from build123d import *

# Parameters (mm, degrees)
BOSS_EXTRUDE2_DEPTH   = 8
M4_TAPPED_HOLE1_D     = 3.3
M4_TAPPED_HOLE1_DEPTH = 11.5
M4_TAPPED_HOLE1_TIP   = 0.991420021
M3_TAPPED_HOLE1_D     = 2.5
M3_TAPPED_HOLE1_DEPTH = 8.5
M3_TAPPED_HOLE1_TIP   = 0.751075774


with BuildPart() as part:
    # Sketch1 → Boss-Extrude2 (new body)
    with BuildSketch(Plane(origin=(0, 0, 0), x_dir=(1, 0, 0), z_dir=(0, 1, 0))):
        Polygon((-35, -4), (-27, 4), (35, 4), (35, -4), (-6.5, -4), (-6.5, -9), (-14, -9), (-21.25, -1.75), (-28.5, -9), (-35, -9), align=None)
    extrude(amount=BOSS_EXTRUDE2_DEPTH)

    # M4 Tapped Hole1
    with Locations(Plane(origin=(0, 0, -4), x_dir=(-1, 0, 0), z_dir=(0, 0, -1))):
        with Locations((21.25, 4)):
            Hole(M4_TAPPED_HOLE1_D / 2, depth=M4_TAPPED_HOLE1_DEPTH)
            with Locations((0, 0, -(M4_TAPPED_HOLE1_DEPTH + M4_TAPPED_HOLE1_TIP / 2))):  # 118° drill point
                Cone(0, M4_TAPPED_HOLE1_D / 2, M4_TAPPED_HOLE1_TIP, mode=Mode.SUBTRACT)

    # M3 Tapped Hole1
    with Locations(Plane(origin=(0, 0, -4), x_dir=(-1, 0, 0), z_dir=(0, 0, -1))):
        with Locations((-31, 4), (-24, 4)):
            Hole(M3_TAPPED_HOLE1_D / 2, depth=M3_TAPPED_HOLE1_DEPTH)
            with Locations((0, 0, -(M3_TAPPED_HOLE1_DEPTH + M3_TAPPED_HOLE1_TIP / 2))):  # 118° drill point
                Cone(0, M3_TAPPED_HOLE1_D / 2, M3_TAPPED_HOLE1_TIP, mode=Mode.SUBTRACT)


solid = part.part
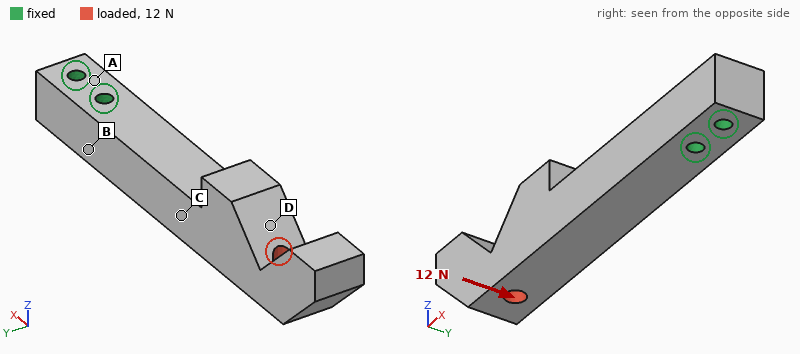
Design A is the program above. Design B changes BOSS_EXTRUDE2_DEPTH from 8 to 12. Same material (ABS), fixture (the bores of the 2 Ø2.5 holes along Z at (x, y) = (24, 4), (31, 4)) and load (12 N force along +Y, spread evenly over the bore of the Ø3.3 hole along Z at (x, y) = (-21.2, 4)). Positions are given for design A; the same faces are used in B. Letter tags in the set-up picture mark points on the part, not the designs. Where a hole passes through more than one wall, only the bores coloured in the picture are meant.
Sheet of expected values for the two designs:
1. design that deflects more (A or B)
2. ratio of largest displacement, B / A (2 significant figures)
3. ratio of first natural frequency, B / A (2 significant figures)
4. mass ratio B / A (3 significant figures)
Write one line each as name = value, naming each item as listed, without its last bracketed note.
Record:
design that deflects more = A
ratio of largest displacement, B / A = 0.35
ratio of first natural frequency, B / A = 1.0
mass ratio B / A = 1.51
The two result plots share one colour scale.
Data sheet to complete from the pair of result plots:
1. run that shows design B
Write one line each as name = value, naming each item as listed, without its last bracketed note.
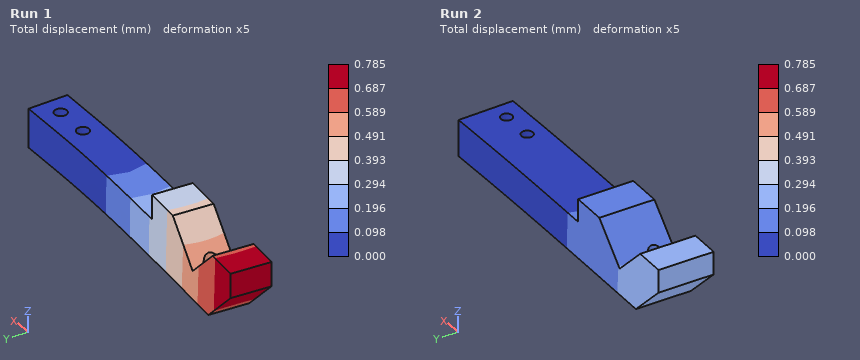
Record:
run that shows design B = Run 2
